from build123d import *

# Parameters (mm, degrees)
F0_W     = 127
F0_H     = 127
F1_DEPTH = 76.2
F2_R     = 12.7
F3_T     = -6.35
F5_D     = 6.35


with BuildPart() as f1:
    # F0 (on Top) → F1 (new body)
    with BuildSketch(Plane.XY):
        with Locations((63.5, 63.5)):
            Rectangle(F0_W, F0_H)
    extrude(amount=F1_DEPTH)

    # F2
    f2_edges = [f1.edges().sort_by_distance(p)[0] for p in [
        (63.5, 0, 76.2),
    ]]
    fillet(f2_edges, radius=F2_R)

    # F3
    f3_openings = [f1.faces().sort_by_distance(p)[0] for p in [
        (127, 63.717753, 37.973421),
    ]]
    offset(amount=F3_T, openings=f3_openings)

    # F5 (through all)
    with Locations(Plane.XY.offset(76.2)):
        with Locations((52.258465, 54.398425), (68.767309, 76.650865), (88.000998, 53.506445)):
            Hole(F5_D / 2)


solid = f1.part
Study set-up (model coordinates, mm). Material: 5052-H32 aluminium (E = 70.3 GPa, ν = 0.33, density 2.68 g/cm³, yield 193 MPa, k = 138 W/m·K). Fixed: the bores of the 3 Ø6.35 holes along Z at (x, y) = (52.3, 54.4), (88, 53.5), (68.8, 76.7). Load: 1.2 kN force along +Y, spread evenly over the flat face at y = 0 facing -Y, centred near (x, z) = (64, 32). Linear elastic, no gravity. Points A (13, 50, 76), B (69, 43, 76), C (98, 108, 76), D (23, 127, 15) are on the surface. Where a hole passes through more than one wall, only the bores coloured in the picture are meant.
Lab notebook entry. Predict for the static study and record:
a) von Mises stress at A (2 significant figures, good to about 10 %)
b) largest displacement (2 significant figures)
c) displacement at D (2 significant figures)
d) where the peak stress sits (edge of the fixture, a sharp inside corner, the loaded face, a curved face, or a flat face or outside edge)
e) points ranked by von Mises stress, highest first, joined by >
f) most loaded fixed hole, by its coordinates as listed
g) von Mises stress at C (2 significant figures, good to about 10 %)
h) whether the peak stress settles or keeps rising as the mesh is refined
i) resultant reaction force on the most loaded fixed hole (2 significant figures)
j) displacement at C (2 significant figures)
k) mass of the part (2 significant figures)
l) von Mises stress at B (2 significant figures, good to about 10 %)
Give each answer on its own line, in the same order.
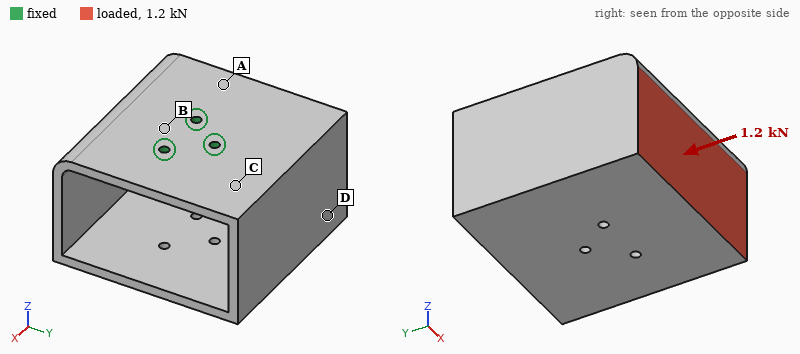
9.1 MPa
0.34 mm
0.27 mm
edge of the fixture
B > C > A > D
(68.8, 76.7)
16 MPa
keeps rising
1.1 kN
0.060 mm
930 g
25 MPa
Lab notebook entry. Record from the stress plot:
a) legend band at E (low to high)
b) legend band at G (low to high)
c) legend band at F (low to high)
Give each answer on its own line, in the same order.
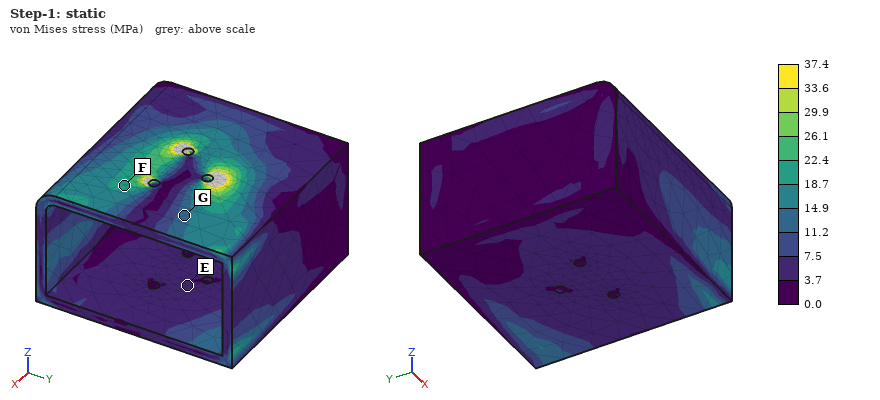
3.7 to 7.5 MPa
11.2 to 14.9 MPa
18.7 to 22.4 MPa
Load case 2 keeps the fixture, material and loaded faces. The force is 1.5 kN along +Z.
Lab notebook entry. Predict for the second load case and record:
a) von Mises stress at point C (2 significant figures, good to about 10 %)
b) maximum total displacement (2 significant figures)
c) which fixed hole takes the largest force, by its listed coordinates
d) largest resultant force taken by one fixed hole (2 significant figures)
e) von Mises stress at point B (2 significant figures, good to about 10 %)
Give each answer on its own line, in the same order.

17 MPa
0.44 mm
(52.3, 54.4)
1.7 kN
54 MPa
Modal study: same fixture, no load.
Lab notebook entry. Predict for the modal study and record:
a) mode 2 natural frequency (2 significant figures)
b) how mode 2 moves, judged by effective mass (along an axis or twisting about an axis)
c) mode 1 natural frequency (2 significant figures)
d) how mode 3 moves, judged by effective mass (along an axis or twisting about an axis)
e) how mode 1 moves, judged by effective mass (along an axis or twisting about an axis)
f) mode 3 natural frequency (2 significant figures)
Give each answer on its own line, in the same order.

430 Hz
along X
350 Hz
along Z
along Y
800 Hz
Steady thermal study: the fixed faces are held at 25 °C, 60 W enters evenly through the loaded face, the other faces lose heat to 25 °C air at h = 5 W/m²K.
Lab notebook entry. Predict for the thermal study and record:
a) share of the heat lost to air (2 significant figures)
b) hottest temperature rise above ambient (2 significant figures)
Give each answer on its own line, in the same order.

15 %
31 K
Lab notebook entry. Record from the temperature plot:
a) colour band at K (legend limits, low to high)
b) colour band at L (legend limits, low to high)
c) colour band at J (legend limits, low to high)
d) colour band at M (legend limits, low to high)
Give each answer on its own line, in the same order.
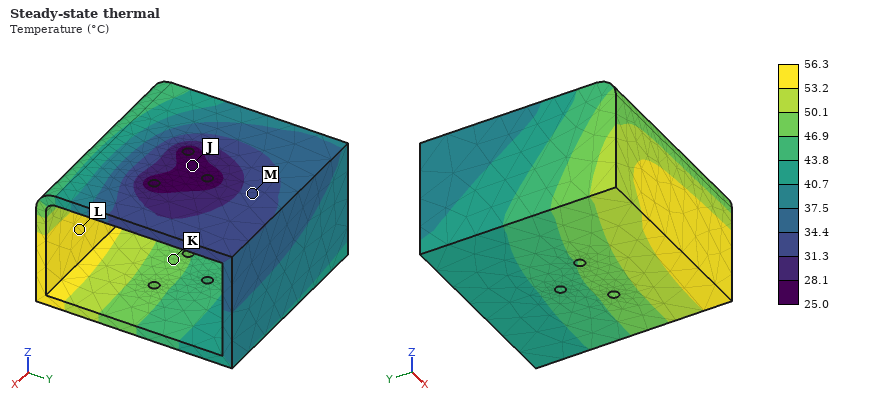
46.9 to 50.1 °C
53.2 to 56.3 °C
25.0 to 28.1 °C
31.3 to 34.4 °C
